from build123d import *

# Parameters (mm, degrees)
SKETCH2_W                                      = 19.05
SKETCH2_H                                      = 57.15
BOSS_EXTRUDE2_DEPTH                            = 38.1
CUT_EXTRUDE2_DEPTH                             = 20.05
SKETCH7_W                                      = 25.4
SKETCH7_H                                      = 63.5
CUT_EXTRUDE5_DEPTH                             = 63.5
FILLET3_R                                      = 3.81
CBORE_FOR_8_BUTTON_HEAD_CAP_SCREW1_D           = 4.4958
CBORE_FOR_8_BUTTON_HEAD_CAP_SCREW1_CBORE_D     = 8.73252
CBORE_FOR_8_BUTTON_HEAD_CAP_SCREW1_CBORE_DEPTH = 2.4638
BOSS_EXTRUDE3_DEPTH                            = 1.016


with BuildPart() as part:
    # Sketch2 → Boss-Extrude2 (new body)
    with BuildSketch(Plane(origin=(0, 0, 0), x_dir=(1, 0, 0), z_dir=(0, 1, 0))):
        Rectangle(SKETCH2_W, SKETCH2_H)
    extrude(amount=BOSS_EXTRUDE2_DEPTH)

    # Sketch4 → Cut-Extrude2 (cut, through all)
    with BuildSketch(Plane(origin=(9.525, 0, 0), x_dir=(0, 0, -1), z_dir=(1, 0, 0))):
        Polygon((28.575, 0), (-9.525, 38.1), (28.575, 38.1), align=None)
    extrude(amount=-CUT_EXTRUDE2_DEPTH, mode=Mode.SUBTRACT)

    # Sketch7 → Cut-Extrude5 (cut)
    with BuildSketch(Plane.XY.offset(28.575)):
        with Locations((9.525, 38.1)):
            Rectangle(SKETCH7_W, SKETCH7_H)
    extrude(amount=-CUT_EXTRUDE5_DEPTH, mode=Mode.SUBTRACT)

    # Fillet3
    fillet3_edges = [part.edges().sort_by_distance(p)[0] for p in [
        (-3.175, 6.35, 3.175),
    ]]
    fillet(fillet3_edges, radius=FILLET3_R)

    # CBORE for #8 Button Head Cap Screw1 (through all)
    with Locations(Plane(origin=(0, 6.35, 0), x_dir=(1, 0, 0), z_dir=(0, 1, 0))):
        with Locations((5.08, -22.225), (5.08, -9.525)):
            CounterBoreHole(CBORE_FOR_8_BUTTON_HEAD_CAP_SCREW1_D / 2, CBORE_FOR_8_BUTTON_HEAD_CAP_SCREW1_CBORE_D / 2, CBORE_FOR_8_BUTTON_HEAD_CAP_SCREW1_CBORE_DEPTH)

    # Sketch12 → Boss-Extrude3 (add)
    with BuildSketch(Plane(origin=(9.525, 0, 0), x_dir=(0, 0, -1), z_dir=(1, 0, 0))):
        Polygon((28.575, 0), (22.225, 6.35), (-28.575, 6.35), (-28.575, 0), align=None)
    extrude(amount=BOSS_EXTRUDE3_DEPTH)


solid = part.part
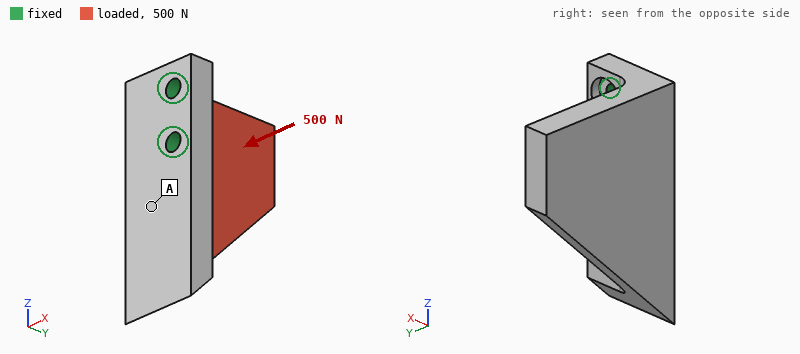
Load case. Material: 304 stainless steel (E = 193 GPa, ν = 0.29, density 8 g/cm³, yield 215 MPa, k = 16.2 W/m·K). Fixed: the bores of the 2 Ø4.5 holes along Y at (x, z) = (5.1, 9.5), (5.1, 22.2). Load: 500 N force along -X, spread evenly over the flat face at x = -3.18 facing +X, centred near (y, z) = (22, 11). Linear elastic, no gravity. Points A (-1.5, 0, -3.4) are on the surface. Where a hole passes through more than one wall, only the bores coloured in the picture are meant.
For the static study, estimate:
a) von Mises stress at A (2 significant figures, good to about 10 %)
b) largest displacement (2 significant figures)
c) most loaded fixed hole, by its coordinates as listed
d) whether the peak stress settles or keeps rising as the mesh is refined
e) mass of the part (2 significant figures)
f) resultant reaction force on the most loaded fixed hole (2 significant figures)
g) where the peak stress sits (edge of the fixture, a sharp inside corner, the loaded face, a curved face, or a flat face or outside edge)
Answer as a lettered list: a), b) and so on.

a) 16 MPa
b) 55 µm
c) (5.1, 9.5)
d) keeps rising
e) 110 g
f) 380 N
g) edge of the fixture
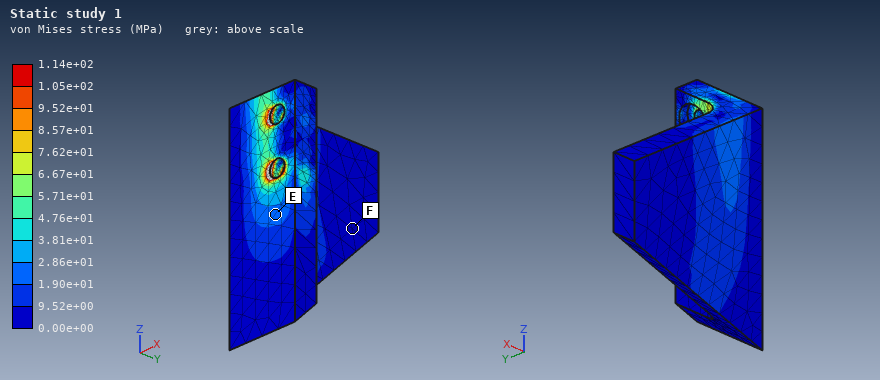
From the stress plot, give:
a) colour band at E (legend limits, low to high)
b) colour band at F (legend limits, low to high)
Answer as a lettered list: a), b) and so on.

a) 1.90e+01 to 2.86e+01 MPa
b) 0.00e+00 to 9.52e+00 MPa
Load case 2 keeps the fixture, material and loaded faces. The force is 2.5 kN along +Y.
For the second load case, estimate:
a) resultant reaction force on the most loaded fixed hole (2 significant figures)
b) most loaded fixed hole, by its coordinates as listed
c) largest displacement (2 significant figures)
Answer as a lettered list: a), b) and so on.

a) 1.9 kN
b) (5.1, 9.5)
c) 44 µm
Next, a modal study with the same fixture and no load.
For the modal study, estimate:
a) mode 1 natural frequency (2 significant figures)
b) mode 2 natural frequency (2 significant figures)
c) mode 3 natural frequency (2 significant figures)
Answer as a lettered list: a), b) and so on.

a) 2600 Hz
b) 3700 Hz
c) 6500 Hz
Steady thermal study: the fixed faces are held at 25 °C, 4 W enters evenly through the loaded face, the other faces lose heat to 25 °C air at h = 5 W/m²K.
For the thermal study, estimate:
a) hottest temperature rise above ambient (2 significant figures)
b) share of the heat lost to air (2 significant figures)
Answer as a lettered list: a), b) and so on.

a) 31 K
b) 9.1 %
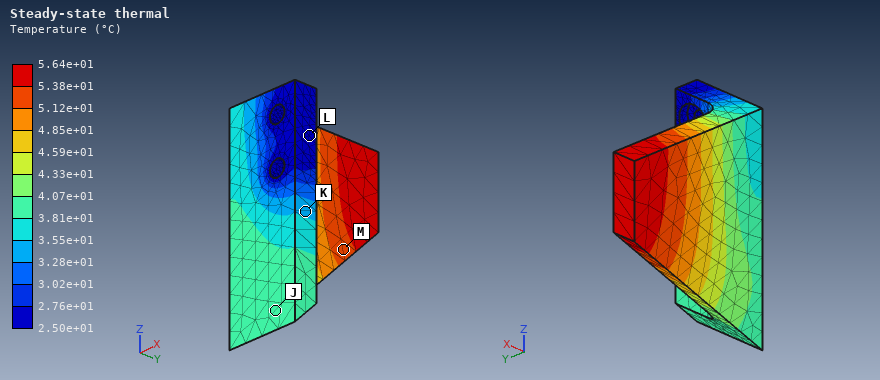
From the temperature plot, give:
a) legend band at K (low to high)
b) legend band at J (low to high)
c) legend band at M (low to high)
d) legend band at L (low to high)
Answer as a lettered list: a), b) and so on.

a) 3.28e+01 to 3.55e+01 °C
b) 3.81e+01 to 4.07e+01 °C
c) 5.12e+01 to 5.38e+01 °C
d) 2.50e+01 to 2.76e+01 °C
